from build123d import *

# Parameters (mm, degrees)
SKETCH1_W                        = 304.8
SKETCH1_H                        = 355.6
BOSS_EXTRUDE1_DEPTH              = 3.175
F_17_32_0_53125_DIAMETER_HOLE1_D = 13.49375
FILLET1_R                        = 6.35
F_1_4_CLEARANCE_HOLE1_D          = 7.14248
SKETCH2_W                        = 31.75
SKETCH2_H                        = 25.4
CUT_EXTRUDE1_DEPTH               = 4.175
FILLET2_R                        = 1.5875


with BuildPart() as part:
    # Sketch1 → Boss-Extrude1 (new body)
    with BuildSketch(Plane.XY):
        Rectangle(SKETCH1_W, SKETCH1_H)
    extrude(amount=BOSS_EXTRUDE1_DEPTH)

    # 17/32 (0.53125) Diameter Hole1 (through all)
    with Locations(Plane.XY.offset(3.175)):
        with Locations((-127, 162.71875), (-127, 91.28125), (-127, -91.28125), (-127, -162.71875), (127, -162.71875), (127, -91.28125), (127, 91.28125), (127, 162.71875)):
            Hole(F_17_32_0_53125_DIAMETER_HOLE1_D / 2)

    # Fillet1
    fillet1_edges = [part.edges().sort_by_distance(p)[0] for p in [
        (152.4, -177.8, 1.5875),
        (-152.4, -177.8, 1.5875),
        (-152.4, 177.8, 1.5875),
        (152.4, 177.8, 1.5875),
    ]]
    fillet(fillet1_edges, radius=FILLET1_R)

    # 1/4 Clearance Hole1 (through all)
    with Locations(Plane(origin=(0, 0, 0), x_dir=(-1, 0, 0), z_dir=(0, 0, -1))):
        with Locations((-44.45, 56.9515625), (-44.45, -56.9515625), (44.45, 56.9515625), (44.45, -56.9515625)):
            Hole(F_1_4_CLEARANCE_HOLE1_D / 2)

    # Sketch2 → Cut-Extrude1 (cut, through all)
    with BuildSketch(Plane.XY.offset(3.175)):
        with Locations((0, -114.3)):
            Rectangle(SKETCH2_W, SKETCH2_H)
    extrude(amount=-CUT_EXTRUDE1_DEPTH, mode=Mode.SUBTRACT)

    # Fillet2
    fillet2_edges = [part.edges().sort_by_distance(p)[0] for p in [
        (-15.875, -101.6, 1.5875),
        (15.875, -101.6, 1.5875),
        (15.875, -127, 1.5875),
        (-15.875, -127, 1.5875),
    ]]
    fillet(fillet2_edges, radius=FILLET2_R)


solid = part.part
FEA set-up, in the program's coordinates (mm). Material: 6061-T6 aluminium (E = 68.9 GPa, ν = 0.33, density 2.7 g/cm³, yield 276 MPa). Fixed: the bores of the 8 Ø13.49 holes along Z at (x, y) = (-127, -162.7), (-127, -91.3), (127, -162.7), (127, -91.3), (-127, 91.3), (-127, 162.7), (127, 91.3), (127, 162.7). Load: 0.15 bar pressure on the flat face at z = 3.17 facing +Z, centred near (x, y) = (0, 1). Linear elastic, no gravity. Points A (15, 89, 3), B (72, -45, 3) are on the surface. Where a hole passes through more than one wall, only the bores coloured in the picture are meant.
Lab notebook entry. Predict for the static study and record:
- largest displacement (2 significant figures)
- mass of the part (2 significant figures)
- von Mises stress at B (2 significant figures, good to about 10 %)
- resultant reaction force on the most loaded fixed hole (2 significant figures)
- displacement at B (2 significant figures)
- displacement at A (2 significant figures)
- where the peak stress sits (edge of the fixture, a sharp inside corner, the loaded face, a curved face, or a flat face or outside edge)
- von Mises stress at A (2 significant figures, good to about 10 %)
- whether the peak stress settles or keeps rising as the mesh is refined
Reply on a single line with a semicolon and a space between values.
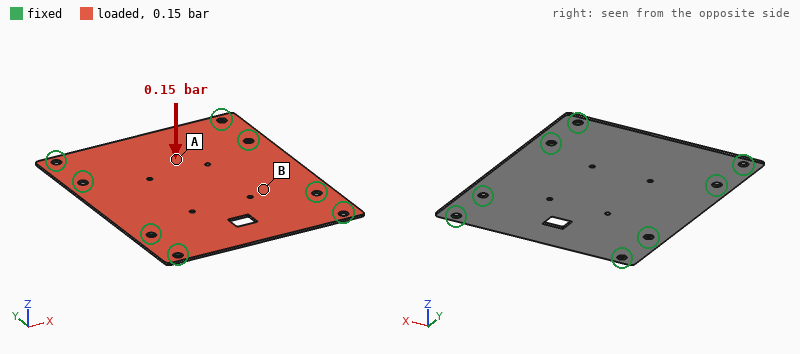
1.2 mm; 910 g; 9.3 MPa; 300 N; 0.67 mm; 0.95 mm; edge of the fixture; 23 MPa; keeps rising
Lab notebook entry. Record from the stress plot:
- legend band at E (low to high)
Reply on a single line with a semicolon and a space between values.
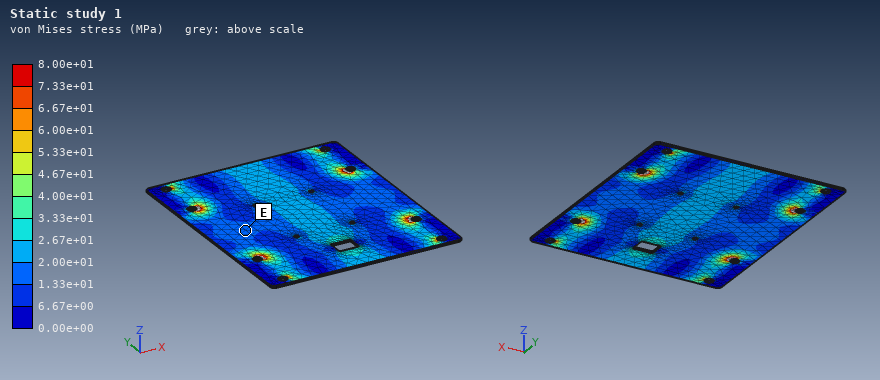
1.33e+01 to 2.00e+01 MPa
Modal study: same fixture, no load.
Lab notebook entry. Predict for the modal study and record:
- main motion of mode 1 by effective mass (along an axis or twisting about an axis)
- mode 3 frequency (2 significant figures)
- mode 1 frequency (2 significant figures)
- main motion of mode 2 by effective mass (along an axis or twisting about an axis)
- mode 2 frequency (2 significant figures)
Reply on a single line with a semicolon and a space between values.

along Z; 360 Hz; 240 Hz; twisting about X; 300 Hz
